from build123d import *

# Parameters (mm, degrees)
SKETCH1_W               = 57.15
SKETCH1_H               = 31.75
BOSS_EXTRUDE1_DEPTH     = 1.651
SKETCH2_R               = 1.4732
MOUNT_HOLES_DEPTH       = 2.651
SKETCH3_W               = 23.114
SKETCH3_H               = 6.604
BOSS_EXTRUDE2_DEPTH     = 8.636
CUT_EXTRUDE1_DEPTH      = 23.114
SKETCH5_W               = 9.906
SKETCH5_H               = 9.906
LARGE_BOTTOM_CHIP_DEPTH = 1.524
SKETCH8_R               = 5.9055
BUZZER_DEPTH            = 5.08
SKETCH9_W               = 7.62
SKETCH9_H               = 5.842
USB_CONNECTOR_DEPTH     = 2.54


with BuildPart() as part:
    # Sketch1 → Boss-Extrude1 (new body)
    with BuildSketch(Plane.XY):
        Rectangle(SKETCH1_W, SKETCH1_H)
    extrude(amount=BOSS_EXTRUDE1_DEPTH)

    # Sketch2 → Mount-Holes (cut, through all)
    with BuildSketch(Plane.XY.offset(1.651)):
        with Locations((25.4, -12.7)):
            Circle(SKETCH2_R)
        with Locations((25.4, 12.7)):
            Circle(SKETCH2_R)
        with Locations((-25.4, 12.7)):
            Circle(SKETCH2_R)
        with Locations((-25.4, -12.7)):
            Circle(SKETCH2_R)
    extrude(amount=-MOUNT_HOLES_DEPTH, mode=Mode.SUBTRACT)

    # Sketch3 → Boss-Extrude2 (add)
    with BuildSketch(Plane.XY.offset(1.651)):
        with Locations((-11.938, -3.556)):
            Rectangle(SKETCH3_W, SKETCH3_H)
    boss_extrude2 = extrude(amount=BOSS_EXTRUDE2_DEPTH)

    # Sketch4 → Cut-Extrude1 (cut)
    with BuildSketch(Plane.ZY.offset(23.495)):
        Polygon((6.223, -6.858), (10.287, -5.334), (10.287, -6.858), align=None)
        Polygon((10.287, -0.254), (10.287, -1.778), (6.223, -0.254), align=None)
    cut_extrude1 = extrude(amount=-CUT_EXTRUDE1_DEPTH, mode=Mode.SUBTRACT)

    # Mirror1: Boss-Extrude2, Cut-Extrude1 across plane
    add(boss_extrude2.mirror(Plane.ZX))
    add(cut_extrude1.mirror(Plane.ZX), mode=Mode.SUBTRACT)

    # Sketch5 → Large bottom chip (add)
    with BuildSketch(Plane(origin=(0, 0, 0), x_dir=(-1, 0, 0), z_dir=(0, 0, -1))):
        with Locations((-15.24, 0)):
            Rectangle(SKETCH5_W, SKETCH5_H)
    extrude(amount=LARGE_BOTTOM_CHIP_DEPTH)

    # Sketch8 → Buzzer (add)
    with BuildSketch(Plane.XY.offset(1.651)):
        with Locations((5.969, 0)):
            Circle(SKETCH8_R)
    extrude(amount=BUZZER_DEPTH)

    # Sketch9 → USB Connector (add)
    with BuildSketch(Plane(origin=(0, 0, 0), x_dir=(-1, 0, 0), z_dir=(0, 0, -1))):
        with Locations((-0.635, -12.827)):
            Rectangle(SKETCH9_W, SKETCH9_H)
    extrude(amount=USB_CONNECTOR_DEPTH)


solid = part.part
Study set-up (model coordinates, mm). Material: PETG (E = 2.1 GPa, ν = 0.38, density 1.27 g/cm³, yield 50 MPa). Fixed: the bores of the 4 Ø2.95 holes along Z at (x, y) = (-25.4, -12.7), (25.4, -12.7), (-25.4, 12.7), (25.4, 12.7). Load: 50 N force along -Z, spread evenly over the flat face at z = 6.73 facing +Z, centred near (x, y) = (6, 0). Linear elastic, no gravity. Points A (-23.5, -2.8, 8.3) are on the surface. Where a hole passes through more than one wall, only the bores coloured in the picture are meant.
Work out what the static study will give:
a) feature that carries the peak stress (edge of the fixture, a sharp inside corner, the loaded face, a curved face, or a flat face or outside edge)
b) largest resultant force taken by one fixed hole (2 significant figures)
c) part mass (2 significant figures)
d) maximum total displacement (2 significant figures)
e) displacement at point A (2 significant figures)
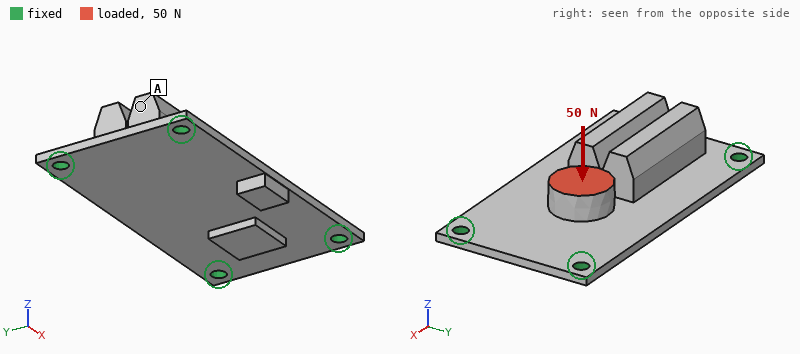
a flat face or outside edge
17 N
7.8 g
0.72 mm
0.20 mm
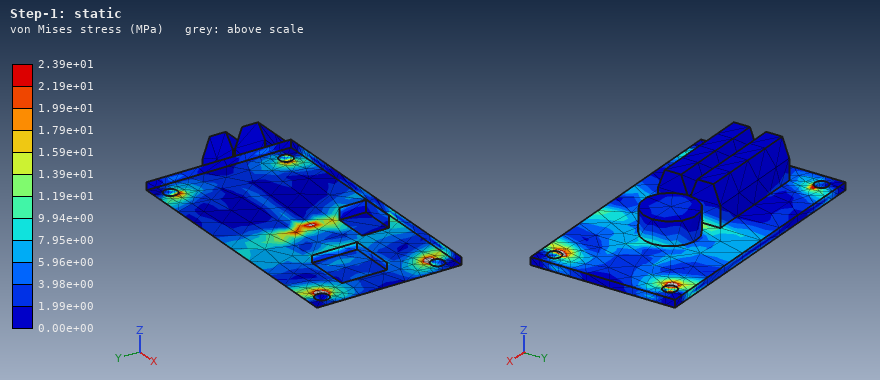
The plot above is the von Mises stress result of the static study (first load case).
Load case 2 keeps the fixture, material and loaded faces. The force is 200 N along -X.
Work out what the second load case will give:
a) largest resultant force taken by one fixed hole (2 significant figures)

62 N
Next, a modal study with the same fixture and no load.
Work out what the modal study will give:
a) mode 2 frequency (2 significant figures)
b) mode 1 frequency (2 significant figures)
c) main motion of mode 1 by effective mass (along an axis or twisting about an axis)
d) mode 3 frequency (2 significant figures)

1700 Hz
710 Hz
along Z
2300 Hz
